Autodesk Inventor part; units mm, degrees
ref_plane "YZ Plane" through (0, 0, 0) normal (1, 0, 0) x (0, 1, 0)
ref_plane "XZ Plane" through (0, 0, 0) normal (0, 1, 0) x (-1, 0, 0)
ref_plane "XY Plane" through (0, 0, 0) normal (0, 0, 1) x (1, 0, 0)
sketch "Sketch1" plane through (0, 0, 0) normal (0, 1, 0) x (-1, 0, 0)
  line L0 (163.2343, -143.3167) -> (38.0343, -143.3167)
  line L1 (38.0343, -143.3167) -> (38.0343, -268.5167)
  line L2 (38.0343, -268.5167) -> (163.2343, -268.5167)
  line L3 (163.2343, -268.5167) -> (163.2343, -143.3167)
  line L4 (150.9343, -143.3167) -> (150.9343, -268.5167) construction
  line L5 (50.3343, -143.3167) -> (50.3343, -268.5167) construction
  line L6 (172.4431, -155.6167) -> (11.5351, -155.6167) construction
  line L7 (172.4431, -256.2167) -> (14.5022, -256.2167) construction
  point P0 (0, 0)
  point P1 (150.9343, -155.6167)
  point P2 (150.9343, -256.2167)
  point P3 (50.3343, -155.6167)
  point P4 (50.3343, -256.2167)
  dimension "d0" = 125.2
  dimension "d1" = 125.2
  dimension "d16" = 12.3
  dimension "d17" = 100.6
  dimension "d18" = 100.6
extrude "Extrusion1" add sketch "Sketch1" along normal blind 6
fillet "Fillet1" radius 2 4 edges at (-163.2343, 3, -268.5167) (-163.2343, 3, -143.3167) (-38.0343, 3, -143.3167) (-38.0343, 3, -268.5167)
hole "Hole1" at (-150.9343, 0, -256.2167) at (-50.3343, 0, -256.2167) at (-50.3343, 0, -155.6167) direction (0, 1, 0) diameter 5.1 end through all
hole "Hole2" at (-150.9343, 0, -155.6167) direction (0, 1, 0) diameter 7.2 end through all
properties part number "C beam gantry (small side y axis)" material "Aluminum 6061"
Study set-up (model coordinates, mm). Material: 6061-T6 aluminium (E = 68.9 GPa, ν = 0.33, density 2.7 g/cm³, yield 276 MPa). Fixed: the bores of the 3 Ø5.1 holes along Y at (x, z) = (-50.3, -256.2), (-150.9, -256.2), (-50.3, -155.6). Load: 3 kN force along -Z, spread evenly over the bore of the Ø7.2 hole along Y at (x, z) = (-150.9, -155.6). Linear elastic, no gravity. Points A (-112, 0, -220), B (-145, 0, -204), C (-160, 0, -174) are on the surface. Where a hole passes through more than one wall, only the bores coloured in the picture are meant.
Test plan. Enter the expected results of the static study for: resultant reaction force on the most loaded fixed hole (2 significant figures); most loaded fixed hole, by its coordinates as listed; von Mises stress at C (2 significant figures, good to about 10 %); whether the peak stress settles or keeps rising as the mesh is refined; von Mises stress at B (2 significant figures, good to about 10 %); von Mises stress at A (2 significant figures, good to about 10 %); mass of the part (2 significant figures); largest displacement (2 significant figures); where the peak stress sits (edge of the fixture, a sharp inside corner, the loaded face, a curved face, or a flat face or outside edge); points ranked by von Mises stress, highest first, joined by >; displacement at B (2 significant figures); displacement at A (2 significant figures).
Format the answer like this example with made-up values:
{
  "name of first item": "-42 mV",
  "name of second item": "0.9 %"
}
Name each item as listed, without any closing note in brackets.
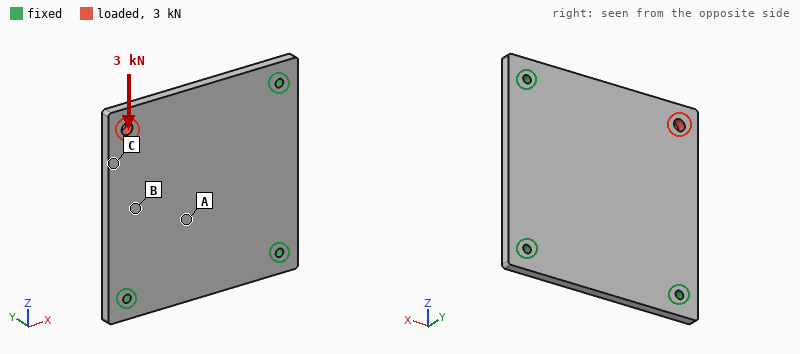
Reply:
{
  "resultant reaction force on the most loaded fixed hole": "2.1 kN",
  "most loaded fixed hole, by its coordinates as listed": "(-150.9, -256.2)",
  "von Mises stress at C": "18 MPa",
  "whether the peak stress settles or keeps rising as the mesh is refined": "keeps rising",
  "von Mises stress at B": "11 MPa",
  "von Mises stress at A": "3.5 MPa",
  "mass of the part": "250 g",
  "largest displacement": "26 µm",
  "where the peak stress sits": "edge of the fixture",
  "points ranked by von Mises stress, highest first, joined by >": "C > B > A",
  "displacement at B": "9.9 µm",
  "displacement at A": "6.0 µm"
}
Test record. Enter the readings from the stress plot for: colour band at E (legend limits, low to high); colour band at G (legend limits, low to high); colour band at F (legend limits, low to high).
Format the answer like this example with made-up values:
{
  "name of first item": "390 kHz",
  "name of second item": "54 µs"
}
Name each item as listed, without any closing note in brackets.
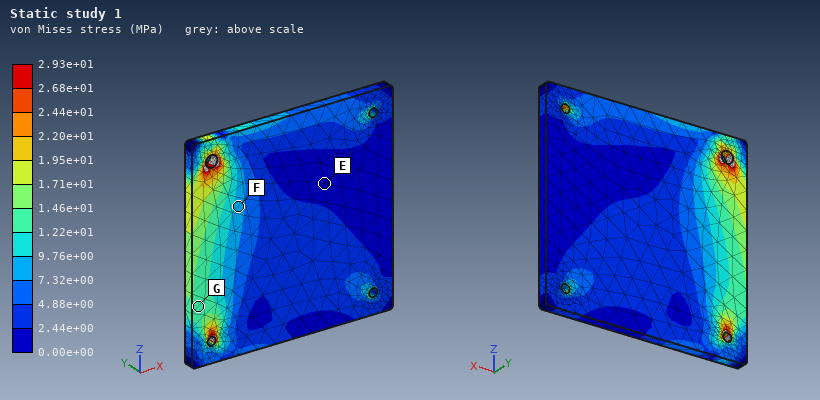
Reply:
{
  "colour band at E": "0.00e+00 to 2.44e+00 MPa",
  "colour band at G": "1.22e+01 to 1.46e+01 MPa",
  "colour band at F": "7.32e+00 to 9.76e+00 MPa"
}
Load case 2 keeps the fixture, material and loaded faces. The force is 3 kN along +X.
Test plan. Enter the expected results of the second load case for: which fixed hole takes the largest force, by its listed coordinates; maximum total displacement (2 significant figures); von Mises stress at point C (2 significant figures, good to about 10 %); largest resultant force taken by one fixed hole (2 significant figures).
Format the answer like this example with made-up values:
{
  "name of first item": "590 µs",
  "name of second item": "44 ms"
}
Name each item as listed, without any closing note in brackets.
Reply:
{
  "which fixed hole takes the largest force, by its listed coordinates": "(-50.3, -155.6)",
  "maximum total displacement": "26 µm",
  "von Mises stress at point C": "6.6 MPa",
  "largest resultant force taken by one fixed hole": "2.1 kN"
}
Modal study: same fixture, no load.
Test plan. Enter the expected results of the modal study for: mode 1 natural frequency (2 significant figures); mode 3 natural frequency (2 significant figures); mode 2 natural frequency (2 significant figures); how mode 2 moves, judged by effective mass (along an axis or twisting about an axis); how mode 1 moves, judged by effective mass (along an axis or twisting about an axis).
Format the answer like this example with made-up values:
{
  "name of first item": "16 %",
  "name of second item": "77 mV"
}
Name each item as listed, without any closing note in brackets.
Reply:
{
  "mode 1 natural frequency": "720 Hz",
  "mode 3 natural frequency": "2600 Hz",
  "mode 2 natural frequency": "2100 Hz",
  "how mode 2 moves, judged by effective mass": "along Y",
  "how mode 1 moves, judged by effective mass": "along Y"
}
